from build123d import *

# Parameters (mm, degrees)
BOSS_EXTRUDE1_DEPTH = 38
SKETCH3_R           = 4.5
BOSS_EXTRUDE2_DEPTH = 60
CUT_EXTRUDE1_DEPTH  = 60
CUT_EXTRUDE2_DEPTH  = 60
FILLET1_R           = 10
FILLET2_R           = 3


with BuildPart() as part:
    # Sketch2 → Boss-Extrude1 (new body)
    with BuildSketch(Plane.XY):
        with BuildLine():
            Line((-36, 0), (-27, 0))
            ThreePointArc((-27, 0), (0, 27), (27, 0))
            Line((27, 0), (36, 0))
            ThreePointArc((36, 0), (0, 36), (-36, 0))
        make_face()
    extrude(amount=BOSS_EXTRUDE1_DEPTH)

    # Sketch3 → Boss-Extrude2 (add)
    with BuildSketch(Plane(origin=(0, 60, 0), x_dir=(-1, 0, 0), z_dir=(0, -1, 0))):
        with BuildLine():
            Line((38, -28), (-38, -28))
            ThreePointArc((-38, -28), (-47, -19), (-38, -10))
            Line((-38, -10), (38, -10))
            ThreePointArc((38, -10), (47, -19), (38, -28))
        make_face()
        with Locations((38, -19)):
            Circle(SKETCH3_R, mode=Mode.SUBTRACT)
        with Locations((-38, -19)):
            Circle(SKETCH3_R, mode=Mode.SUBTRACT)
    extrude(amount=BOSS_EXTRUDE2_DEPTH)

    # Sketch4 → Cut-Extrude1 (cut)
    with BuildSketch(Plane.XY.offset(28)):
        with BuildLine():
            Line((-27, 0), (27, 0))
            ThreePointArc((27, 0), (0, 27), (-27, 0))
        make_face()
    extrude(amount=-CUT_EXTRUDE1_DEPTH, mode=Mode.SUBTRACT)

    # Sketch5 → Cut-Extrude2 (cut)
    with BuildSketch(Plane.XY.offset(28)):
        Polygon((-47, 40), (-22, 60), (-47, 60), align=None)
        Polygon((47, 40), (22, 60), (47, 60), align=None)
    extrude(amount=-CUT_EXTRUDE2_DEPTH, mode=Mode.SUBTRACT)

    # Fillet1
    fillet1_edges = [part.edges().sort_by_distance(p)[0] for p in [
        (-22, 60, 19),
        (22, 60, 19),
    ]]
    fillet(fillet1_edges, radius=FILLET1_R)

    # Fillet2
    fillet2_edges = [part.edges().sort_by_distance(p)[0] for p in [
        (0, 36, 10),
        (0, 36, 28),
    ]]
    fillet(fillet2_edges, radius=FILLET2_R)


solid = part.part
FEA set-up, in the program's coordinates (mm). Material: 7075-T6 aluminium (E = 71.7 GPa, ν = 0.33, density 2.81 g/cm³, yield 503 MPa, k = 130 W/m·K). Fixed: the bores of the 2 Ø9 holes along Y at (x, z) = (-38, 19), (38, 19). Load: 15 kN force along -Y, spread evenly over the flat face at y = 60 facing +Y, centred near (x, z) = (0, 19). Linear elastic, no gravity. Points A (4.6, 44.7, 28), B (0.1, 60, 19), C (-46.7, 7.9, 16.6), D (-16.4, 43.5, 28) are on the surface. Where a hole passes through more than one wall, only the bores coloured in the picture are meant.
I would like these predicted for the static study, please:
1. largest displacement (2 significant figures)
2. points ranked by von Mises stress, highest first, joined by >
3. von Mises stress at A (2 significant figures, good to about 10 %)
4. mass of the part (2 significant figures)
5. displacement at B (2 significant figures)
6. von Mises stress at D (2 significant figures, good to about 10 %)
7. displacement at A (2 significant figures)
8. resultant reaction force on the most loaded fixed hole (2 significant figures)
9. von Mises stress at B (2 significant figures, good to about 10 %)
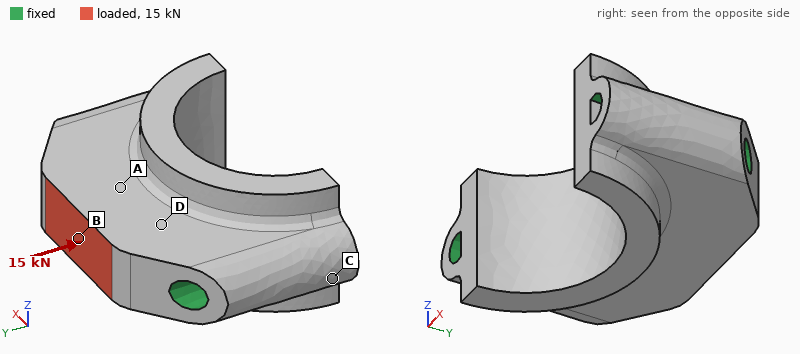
17 µm
B > D > A > C
16 MPa
230 g
16 µm
21 MPa
13 µm
8.7 kN
26 MPa
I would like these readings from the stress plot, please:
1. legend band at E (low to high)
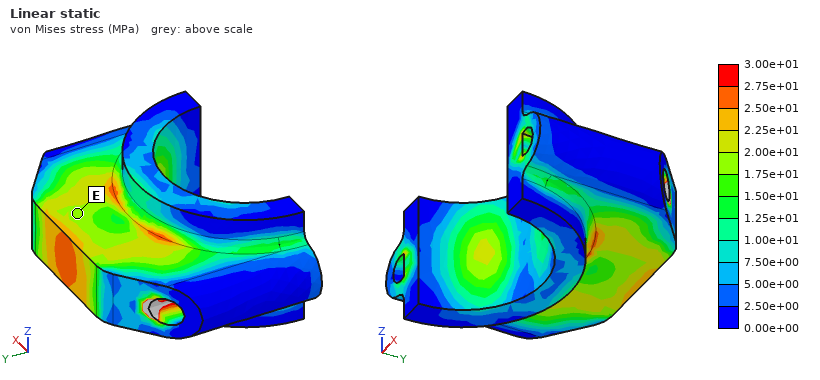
1.75e+01 to 2.00e+01 MPa
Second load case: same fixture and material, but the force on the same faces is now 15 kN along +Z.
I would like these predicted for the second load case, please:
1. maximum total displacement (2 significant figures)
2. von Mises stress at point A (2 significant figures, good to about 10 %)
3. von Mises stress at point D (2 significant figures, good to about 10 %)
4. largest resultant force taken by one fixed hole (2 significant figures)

0.11 mm
73 MPa
76 MPa
7.5 kN
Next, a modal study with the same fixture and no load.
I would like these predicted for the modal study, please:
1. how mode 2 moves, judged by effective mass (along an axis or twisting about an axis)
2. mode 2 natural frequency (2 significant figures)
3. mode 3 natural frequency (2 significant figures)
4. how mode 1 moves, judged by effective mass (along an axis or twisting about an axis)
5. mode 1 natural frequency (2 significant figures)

along Y
18 kHz
19 kHz
along Z
12 kHz
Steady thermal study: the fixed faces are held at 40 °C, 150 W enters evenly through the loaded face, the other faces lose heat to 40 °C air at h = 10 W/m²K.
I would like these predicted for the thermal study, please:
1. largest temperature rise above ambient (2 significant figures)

42 K
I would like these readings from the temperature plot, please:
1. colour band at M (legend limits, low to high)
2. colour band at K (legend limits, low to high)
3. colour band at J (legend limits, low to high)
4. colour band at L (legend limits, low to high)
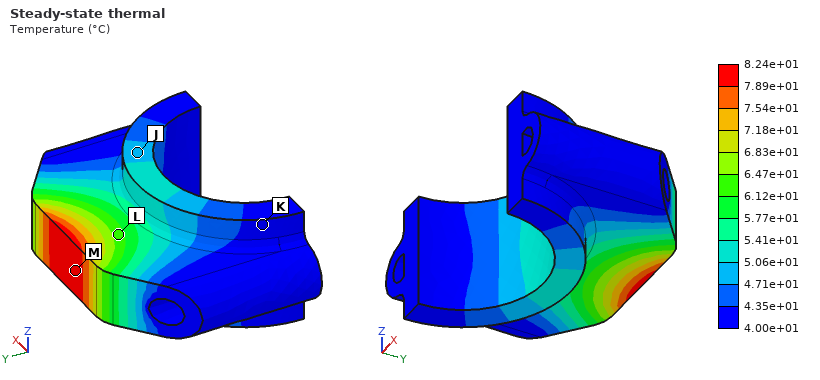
7.89e+01 to 8.24e+01 °C
4.00e+01 to 4.35e+01 °C
4.71e+01 to 5.06e+01 °C
6.12e+01 to 6.47e+01 °C
